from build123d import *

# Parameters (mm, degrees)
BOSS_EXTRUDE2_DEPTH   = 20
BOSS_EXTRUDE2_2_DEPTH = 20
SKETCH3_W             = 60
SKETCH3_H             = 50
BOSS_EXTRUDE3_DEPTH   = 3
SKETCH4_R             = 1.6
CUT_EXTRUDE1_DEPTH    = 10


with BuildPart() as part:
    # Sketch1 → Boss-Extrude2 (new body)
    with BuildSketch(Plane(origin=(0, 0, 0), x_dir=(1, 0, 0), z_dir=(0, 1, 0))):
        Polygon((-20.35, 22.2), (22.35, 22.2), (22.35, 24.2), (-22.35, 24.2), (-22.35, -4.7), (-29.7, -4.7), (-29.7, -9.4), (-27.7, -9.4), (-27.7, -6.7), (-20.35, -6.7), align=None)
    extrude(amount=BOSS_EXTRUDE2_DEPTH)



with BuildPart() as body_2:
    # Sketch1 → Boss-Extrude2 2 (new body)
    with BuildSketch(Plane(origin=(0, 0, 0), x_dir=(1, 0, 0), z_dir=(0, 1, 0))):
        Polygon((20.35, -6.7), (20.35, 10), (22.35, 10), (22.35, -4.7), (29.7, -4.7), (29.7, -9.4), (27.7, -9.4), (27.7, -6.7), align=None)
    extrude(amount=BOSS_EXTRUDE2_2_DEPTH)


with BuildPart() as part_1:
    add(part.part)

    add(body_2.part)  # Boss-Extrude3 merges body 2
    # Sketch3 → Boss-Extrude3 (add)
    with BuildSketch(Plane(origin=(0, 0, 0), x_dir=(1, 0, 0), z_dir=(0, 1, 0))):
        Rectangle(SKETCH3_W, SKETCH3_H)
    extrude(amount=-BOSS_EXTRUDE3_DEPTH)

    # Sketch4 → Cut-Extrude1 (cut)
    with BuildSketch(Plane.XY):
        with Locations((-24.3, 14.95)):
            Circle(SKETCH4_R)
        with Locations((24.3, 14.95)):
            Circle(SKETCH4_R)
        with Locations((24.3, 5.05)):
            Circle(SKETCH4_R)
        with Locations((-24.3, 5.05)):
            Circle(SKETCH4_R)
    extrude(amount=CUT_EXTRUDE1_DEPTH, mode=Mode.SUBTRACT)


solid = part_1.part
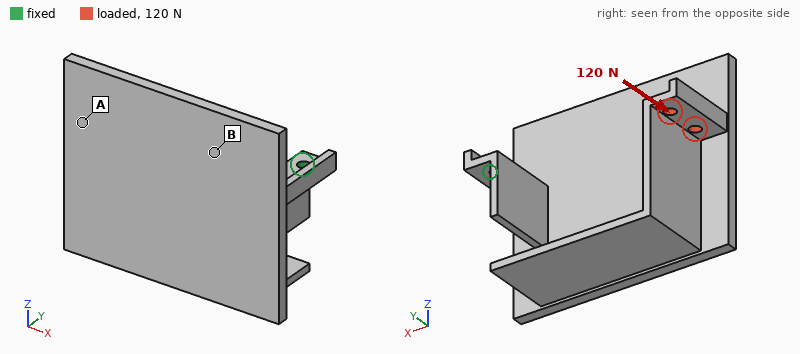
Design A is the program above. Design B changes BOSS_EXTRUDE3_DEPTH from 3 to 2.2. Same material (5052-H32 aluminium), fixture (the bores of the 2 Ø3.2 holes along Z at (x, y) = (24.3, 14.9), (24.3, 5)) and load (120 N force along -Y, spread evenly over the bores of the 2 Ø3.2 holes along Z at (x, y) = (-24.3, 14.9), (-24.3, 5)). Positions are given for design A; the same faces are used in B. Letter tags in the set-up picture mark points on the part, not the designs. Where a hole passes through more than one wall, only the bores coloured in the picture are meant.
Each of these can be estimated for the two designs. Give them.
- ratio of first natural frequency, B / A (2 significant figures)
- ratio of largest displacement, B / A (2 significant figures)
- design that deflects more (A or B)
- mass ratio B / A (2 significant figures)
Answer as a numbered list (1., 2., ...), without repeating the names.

1. 0.79
2. 1.9
3. B
4. 0.82
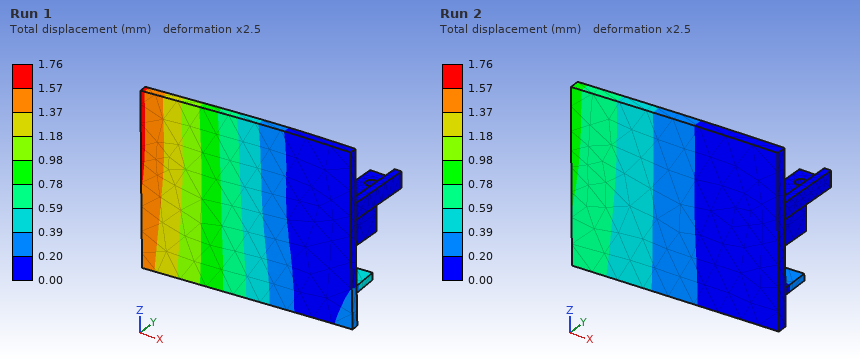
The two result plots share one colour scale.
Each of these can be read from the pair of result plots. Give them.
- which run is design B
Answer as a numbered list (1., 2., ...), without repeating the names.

1. Run 1
